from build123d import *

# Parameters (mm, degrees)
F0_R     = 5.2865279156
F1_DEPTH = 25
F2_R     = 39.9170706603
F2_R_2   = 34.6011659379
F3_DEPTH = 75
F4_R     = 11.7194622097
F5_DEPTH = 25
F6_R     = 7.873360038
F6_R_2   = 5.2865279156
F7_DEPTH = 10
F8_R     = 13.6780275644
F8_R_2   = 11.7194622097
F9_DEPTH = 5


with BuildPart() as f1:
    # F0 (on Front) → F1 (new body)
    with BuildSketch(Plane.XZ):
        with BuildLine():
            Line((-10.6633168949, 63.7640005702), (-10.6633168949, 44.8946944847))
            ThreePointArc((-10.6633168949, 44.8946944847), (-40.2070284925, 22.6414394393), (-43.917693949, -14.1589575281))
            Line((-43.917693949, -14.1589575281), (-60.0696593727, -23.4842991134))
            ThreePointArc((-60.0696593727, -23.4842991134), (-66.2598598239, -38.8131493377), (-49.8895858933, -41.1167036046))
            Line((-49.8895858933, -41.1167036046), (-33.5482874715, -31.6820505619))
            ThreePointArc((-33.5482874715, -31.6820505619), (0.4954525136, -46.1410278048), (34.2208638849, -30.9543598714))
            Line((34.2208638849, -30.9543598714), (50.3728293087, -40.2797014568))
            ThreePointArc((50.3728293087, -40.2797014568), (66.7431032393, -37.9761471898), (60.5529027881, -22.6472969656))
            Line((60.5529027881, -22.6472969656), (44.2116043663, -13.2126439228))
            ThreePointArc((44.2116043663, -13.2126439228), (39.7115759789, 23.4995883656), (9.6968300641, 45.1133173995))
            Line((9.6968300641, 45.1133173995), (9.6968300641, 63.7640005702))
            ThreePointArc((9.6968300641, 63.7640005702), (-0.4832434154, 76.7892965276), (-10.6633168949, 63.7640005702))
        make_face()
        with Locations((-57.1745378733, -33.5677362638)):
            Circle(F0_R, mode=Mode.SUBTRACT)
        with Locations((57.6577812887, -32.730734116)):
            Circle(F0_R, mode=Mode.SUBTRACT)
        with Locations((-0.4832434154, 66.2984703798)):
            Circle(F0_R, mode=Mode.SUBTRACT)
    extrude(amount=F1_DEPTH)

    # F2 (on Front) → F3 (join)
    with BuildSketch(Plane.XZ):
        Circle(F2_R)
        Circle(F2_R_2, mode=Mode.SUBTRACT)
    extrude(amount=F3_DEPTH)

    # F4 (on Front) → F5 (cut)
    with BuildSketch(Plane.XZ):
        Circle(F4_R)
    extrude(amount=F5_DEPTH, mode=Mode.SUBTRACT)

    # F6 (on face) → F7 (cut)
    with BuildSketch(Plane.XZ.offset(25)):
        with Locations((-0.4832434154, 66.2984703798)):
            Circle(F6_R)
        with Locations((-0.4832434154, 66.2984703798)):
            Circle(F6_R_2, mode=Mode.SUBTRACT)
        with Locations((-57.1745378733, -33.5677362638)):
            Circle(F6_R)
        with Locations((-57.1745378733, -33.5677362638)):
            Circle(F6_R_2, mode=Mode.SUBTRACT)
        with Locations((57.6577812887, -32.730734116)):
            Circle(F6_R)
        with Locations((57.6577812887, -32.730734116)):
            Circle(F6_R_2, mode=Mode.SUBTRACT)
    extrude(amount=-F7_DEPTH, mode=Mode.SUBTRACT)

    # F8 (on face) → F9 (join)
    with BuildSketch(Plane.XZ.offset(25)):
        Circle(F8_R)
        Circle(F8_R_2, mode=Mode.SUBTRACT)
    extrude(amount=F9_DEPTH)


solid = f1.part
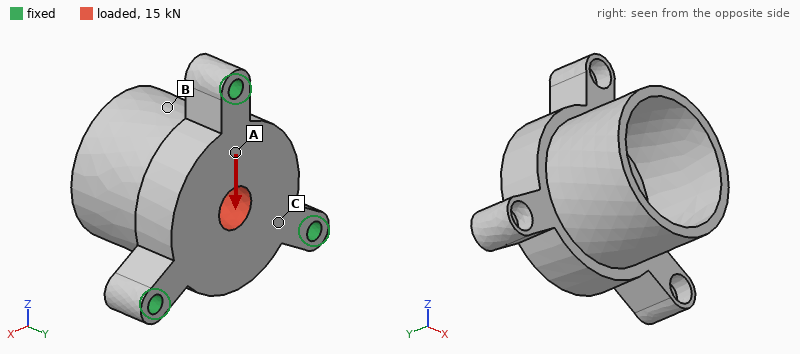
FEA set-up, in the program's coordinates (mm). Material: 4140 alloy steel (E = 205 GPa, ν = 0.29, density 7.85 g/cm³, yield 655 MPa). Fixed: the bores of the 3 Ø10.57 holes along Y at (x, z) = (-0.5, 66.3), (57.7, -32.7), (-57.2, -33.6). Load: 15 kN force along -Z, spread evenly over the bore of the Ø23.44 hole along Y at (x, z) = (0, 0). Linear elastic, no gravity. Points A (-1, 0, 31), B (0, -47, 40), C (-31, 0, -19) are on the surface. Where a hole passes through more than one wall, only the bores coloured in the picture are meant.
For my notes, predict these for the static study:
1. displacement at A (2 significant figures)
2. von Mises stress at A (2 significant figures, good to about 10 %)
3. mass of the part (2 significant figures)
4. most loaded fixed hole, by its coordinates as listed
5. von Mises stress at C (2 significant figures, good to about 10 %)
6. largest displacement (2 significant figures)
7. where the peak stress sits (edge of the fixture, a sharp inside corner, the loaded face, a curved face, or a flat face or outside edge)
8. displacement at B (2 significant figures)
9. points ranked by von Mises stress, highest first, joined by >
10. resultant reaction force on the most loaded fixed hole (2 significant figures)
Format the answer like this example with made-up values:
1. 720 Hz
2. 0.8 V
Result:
1. 2.6 µm
2. 12 MPa
3. 2.0 kg
4. (-0.5, 66.3)
5. 6.9 MPa
6. 9.1 µm
7. edge of the fixture
8. 1.9 µm
9. A > C > B
10. 7.9 kN
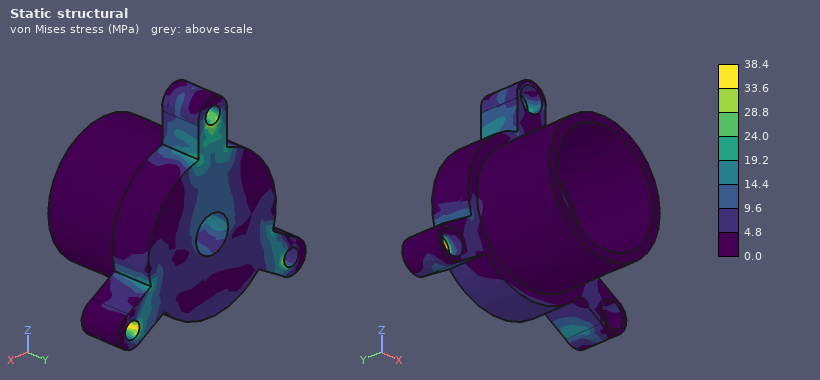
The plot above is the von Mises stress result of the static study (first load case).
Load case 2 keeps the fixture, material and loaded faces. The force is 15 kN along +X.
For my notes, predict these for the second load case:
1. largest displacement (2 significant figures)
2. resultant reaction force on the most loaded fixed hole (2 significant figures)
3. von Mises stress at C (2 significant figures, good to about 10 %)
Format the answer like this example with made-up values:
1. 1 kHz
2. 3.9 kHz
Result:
1. 8.3 µm
2. 6.9 kN
3. 11 MPa
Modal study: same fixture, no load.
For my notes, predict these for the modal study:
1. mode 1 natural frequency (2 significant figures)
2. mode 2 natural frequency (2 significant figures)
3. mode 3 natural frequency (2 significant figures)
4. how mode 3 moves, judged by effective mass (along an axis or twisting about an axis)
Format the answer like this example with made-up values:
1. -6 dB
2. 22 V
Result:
1. 4100 Hz
2. 4100 Hz
3. 4700 Hz
4. along Y
